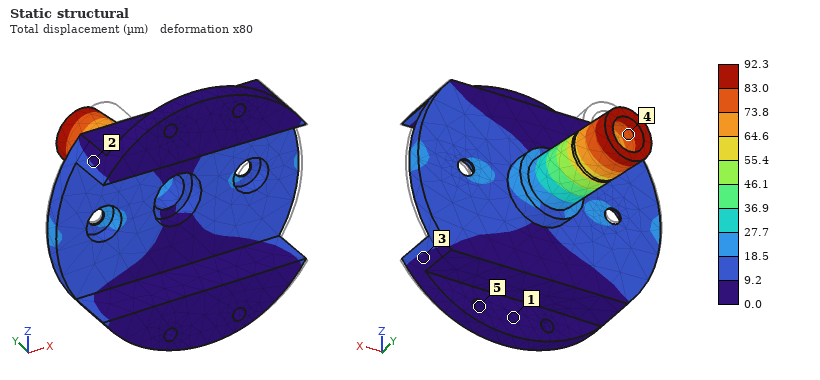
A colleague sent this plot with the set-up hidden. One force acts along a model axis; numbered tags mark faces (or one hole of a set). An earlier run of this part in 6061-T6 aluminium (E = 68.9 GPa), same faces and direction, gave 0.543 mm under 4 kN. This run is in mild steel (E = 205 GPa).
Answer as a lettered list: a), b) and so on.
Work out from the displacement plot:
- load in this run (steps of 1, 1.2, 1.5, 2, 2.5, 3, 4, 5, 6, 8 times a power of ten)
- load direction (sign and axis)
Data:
a) 2 kN
b) -X
